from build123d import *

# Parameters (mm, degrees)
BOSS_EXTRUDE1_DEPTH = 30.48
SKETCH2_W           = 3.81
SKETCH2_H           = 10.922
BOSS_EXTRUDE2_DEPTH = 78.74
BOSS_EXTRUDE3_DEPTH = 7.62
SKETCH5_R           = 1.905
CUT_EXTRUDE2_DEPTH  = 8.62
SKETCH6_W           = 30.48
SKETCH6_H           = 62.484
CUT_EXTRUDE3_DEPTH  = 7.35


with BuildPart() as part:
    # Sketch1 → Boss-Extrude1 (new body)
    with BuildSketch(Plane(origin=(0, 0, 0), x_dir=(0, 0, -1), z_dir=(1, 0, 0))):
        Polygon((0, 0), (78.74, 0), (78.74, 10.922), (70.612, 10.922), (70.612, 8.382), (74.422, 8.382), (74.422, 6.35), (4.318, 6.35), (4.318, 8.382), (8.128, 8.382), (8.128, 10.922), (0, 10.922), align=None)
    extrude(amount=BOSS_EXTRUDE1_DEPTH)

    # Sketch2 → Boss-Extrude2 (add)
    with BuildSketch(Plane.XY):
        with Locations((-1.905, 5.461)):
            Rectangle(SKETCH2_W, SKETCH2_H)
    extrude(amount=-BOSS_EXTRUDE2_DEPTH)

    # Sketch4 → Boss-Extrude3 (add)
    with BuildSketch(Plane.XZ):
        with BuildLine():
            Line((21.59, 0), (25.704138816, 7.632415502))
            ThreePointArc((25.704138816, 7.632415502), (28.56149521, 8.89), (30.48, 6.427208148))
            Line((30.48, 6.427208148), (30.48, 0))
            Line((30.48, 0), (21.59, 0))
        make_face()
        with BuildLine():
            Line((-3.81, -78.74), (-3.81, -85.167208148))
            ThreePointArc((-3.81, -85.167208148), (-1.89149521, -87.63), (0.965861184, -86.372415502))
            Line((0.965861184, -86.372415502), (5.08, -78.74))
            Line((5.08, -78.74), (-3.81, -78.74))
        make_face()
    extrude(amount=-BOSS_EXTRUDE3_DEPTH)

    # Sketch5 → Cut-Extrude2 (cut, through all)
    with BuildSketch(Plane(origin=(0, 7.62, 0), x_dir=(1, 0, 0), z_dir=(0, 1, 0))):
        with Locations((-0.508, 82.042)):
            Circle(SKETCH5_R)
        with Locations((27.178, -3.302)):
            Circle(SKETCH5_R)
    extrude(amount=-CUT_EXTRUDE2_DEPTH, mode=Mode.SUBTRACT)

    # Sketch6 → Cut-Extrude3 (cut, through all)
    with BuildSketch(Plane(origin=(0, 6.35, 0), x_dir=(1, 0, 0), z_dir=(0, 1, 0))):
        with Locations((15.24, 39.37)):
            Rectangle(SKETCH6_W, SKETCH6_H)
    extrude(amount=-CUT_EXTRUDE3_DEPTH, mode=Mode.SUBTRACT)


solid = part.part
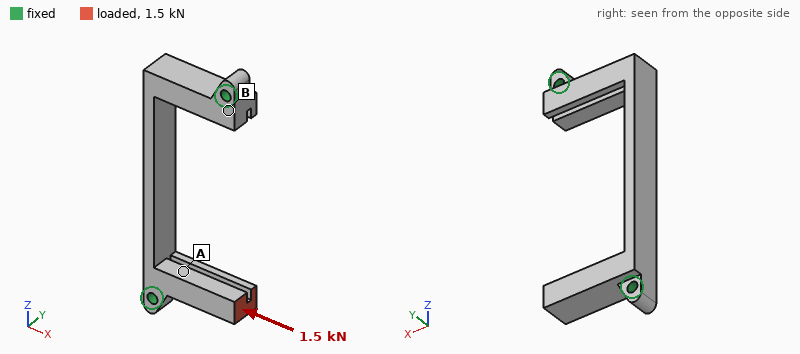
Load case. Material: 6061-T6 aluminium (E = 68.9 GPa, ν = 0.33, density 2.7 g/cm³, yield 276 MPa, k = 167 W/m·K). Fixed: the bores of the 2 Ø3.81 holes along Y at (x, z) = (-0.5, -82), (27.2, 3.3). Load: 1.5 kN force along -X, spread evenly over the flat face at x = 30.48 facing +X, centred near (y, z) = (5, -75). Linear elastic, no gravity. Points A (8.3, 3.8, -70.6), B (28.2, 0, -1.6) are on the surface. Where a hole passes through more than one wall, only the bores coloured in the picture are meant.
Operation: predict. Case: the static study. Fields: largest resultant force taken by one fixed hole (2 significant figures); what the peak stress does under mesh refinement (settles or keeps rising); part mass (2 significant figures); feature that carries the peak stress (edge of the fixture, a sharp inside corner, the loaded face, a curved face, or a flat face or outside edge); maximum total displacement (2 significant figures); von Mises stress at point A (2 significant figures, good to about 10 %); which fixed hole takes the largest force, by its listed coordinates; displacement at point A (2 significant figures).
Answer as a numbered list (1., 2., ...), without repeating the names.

1. 1.5 kN
2. keeps rising
3. 24 g
4. edge of the fixture
5. 82 µm
6. 20 MPa
7. (-0.5, -82)
8. 33 µm
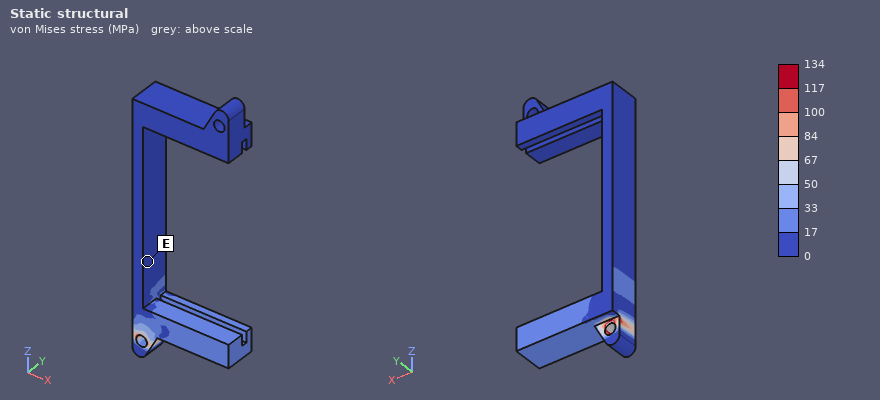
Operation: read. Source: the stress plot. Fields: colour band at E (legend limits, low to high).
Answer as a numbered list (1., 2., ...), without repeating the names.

1. 0 to 17 MPa
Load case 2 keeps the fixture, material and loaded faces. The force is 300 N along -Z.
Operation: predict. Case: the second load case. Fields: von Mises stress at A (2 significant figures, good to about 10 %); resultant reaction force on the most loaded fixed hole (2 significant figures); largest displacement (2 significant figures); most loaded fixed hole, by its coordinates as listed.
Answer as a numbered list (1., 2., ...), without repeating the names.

1. 67 MPa
2. 330 N
3. 0.16 mm
4. (-0.5, -82)
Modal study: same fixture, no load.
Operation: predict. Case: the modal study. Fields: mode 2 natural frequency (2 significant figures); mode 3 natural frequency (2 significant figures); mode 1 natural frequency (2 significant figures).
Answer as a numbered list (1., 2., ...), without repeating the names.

1. 4000 Hz
2. 5300 Hz
3. 3800 Hz
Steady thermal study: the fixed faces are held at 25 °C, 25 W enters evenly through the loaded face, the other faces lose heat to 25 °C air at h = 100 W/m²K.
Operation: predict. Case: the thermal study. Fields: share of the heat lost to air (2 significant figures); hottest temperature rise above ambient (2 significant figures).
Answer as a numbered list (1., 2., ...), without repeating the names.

1. 20 %
2. 56 K
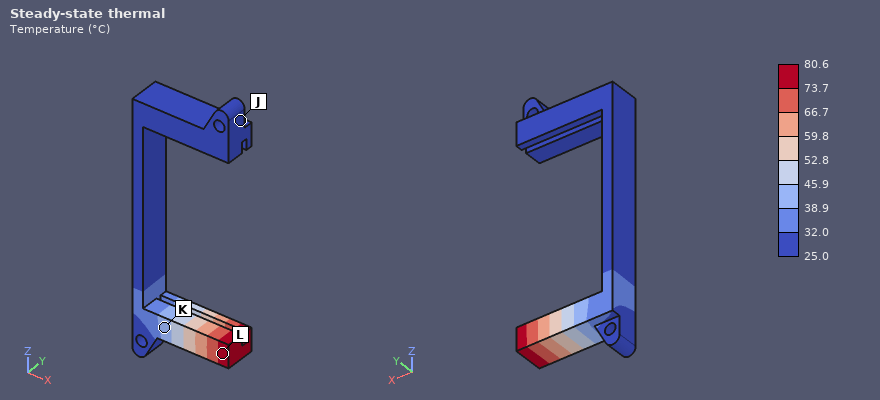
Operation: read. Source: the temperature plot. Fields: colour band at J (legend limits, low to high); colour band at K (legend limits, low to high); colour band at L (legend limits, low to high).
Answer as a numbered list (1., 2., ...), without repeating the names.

1. 25.0 to 32.0 °C
2. 38.9 to 45.9 °C
3. 73.7 to 80.6 °C
